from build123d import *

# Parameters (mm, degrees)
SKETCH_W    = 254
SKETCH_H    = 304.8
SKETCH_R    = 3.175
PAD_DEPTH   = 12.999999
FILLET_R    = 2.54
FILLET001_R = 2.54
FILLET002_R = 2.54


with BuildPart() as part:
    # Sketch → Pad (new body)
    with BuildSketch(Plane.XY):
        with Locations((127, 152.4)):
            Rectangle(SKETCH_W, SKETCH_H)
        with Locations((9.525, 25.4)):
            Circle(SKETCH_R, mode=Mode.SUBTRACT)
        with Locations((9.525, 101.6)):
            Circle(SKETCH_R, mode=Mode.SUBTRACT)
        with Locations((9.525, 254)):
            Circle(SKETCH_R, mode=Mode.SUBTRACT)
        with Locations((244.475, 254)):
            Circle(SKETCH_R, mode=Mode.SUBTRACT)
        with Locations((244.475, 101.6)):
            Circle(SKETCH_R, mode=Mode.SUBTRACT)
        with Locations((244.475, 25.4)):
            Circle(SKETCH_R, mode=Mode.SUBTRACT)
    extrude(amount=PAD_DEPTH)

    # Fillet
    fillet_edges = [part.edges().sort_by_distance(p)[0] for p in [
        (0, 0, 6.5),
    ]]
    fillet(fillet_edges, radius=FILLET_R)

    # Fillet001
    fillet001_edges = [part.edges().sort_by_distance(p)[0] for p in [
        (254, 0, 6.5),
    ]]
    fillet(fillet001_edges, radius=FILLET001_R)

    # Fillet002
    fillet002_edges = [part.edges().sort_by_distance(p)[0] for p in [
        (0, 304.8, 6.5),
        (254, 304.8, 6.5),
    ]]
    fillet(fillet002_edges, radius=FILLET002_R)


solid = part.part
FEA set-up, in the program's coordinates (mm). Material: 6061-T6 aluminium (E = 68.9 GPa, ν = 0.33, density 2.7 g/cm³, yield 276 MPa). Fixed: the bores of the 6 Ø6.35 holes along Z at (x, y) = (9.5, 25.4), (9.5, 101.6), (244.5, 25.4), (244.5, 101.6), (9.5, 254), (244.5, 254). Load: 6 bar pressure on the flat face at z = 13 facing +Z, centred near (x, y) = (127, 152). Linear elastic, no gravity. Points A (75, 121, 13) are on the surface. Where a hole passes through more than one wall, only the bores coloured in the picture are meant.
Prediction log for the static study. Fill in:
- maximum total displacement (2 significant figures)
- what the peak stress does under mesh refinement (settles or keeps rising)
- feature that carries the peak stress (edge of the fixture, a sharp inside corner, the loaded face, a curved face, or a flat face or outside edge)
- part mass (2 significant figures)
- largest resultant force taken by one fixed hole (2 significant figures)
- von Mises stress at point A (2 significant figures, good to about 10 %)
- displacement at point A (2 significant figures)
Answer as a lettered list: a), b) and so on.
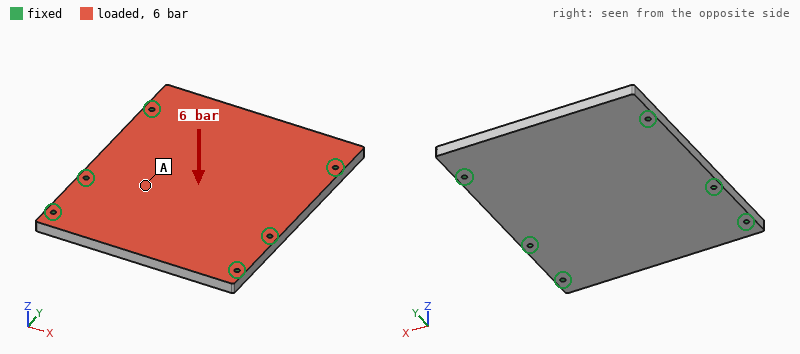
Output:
a) 0.76 mm
b) keeps rising
c) edge of the fixture
d) 2.7 kg
e) 9.9 kN
f) 36 MPa
g) 0.47 mm
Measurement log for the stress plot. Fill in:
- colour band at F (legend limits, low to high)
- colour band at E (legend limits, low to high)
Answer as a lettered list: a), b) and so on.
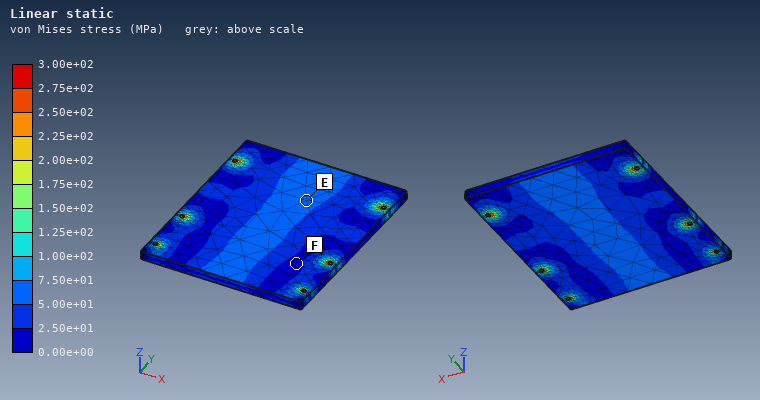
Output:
a) 0.00e+00 to 2.50e+01 MPa
b) 5.00e+01 to 7.50e+01 MPa
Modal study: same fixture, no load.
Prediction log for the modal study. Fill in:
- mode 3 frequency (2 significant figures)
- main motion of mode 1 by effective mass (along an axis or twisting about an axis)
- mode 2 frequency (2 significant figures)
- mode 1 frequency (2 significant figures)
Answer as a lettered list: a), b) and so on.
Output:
a) 1500 Hz
b) along Z
c) 1100 Hz
d) 910 Hz
